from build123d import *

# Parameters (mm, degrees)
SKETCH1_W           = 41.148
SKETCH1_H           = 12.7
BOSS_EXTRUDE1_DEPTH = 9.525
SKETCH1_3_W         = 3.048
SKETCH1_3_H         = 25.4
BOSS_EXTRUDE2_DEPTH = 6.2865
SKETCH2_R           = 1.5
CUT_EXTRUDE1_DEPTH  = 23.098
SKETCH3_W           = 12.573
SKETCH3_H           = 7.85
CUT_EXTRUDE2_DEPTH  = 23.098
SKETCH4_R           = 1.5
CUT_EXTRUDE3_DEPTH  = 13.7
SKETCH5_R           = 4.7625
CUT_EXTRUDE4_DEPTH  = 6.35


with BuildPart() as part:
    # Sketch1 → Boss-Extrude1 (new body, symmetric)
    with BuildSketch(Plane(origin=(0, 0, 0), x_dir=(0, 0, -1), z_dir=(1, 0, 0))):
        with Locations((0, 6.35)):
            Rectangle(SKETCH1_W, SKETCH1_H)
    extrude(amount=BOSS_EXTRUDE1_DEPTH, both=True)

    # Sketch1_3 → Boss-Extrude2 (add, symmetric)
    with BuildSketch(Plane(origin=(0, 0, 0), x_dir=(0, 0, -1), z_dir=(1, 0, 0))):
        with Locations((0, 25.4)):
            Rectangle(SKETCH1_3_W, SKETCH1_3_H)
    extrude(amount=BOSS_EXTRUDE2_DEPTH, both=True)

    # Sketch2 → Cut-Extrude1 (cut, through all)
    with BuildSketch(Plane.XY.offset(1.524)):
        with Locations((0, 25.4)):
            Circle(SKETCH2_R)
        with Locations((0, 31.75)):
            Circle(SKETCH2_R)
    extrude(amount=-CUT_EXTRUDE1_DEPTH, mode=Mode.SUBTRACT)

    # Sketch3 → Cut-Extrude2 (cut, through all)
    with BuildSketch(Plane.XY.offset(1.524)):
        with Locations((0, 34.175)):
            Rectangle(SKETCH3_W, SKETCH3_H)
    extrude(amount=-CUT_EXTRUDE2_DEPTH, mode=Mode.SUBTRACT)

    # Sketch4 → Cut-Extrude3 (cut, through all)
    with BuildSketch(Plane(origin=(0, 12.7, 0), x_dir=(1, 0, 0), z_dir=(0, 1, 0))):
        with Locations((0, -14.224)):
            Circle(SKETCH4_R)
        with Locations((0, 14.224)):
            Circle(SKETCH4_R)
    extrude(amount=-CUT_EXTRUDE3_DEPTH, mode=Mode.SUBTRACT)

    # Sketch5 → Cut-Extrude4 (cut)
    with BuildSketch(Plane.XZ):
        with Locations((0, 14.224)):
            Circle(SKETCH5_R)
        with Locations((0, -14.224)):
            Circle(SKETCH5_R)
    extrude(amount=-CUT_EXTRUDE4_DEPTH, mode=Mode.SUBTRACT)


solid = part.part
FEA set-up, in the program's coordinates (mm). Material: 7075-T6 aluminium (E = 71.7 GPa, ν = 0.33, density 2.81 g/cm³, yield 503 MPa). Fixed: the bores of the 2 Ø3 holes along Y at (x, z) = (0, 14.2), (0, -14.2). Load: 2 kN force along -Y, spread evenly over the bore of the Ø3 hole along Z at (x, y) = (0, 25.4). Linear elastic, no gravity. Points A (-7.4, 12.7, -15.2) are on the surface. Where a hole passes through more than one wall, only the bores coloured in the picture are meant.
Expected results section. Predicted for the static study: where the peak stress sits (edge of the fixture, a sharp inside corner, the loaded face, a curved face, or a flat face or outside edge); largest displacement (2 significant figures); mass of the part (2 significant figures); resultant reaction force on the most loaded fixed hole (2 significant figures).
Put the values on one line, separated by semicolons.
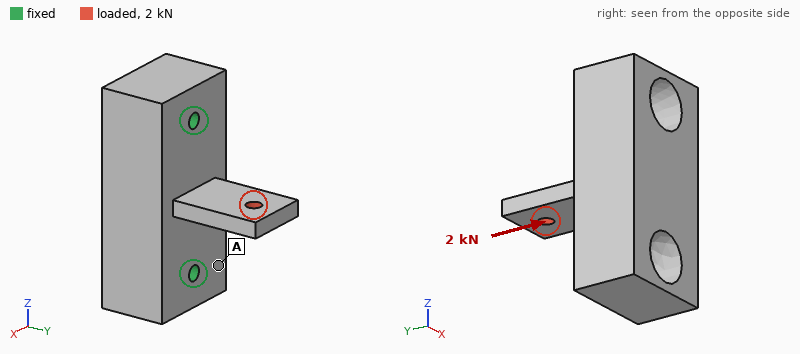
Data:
the loaded face; 22 µm; 27 g; 1.1 kN
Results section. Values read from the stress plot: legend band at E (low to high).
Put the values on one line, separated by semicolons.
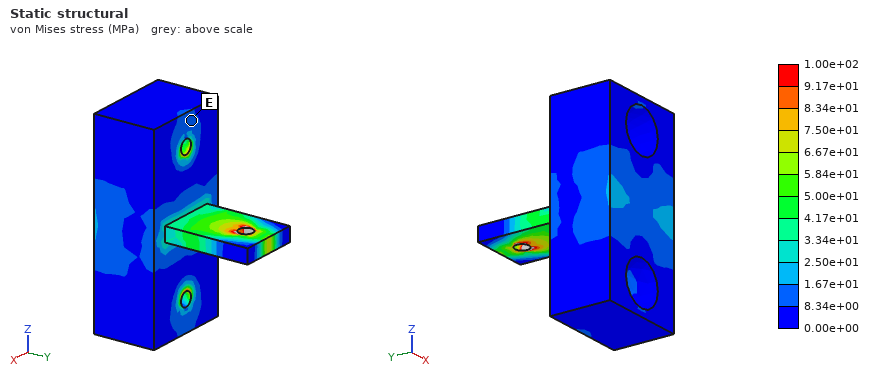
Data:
8.34e+00 to 1.67e+01 MPa
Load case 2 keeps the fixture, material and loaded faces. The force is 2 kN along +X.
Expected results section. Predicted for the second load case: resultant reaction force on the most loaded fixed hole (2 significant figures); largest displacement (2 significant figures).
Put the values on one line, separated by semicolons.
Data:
1.0 kN; 0.19 mm
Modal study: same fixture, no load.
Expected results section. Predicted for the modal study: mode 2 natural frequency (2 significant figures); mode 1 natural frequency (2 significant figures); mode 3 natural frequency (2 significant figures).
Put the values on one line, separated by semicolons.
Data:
13 kHz; 7500 Hz; 21 kHz
